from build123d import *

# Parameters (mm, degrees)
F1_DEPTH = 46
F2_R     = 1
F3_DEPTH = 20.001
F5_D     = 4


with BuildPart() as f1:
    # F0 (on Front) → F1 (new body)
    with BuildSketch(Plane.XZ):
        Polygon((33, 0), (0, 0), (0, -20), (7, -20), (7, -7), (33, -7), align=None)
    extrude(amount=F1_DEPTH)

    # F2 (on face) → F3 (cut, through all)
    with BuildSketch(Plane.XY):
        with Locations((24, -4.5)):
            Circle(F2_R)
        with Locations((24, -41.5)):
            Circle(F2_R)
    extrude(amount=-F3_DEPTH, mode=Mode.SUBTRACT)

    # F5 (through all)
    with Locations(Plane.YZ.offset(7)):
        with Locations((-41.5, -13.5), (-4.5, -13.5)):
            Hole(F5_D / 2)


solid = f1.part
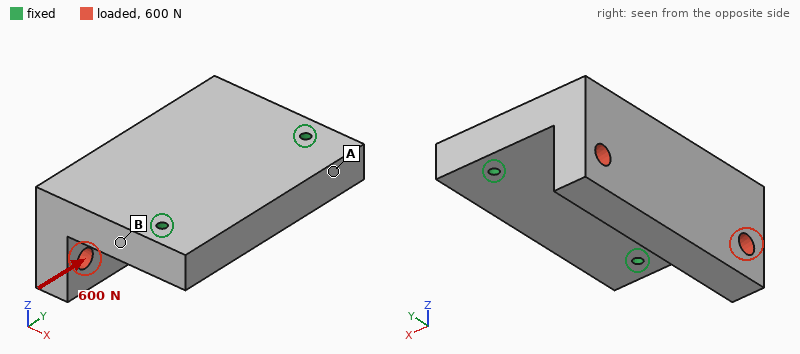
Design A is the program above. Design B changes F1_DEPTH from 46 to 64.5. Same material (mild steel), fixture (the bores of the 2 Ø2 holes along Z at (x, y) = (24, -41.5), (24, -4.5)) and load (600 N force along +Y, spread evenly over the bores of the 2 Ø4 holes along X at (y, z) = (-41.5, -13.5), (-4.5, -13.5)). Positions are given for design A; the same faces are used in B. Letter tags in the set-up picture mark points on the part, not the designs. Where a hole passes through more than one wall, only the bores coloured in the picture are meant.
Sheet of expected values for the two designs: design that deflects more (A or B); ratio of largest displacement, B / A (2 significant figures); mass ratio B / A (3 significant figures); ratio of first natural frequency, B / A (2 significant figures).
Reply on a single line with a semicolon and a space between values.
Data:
B; 1.1; 1.41; 0.89
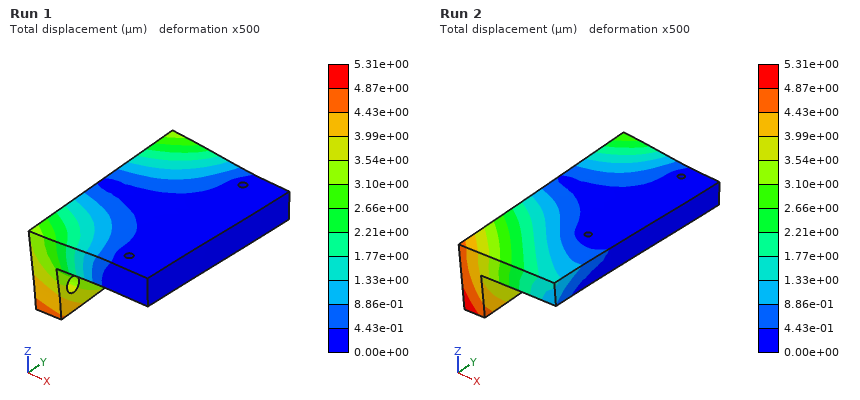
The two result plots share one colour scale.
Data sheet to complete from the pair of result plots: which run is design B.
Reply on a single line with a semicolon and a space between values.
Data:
Run 2
